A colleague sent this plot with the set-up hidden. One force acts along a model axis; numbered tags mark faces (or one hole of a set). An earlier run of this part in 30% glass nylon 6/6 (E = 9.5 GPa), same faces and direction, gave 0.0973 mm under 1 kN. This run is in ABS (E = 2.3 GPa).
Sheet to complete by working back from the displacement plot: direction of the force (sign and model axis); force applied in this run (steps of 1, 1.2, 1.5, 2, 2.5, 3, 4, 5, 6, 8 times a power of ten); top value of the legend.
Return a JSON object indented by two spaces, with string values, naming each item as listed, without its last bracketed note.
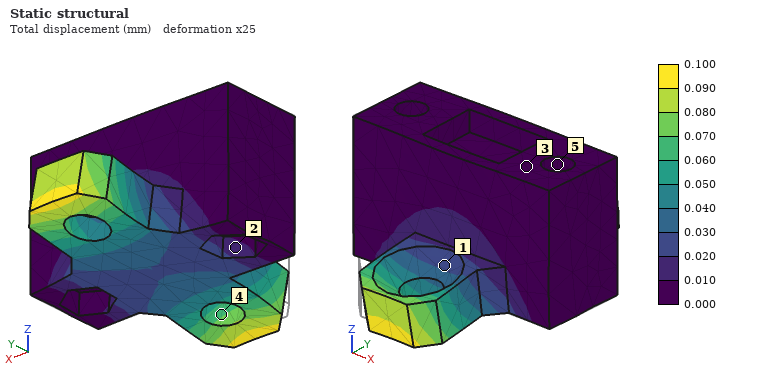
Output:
{
  "direction of the force": "+Y",
  "force applied in this run": "250 N",
  "top value of the legend": "0.100 mm"
}
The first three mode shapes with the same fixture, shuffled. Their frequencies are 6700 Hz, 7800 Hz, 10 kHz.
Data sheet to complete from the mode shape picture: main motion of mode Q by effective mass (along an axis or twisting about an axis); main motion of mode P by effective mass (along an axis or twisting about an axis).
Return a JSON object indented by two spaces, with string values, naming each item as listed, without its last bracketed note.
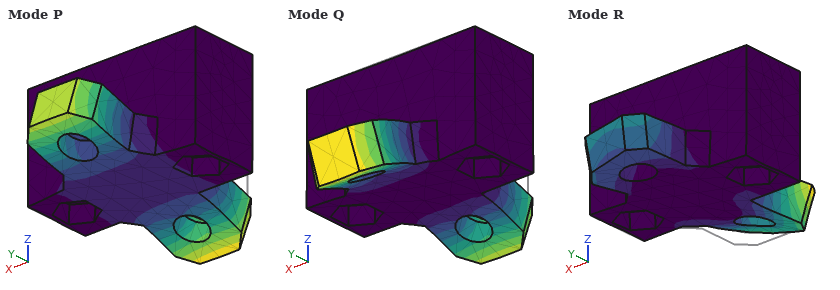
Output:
{
  "main motion of mode Q by effective mass": "along Z",
  "main motion of mode P by effective mass": "twisting about X"
}
